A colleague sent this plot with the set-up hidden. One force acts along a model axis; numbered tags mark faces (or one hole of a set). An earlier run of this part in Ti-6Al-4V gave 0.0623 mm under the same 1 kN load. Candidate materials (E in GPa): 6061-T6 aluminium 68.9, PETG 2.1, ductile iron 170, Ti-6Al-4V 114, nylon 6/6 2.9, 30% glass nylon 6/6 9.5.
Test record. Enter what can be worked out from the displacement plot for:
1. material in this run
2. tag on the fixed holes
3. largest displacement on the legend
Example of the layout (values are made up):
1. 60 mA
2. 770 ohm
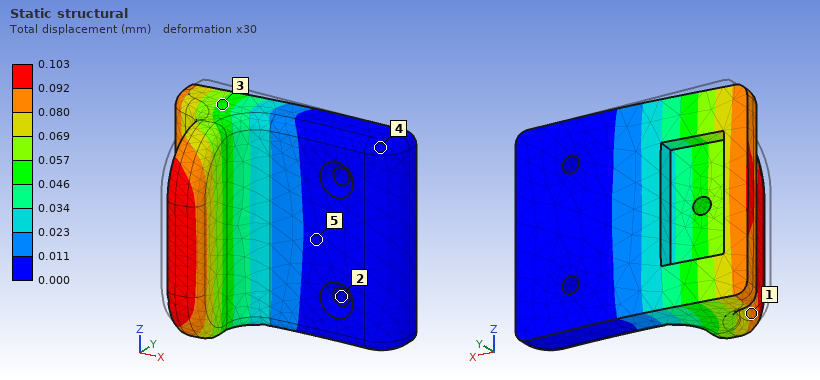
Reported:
1. 6061-T6 aluminium
2. 2
3. 0.103 mm
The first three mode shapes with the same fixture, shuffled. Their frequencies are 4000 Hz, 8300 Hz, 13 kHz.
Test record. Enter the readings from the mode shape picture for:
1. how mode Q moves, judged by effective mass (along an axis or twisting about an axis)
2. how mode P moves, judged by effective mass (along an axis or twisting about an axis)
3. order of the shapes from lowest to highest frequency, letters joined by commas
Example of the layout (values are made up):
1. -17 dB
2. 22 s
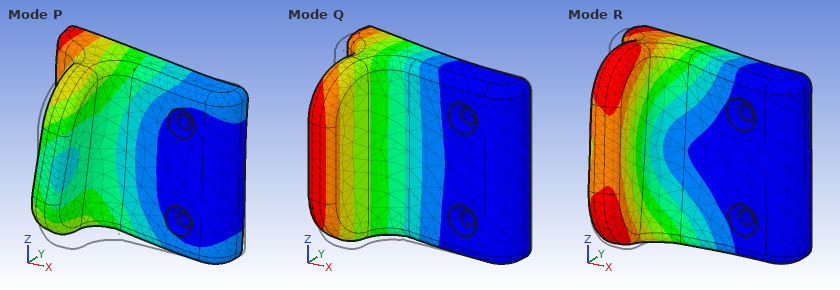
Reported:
1. along Y
2. along Z
3. Q, R, P
